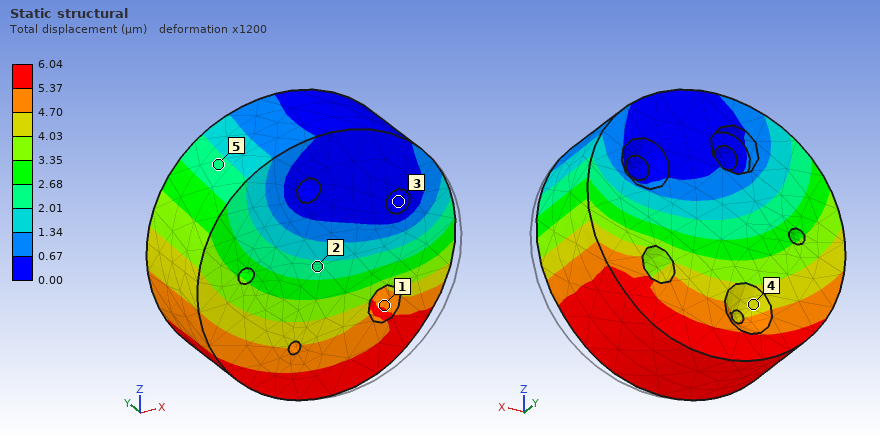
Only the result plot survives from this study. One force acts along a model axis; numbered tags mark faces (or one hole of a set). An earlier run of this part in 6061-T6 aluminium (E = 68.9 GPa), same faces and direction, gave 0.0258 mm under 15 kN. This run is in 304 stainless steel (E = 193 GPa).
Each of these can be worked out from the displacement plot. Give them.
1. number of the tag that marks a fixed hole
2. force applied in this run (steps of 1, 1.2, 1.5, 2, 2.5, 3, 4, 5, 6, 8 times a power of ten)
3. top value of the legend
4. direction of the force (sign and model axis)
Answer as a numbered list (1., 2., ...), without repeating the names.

1. 3
2. 10 kN
3. 6.04 µm
4. -X
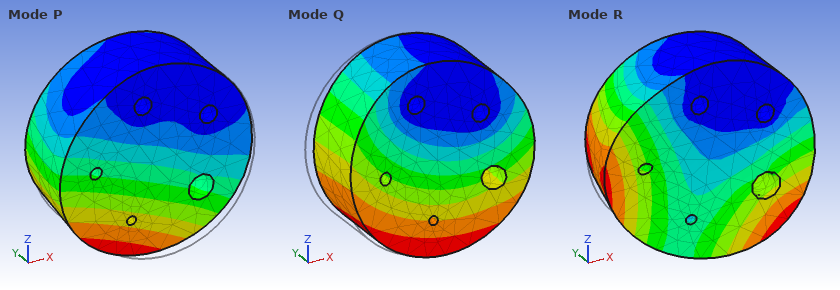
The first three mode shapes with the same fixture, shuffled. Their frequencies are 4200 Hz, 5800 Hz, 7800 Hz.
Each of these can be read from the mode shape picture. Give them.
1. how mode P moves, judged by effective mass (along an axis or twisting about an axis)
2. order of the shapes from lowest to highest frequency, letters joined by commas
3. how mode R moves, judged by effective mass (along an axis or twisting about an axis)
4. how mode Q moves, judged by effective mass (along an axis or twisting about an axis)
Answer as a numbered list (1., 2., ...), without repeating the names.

1. along Y
2. P, Q, R
3. twisting about Z
4. along X
